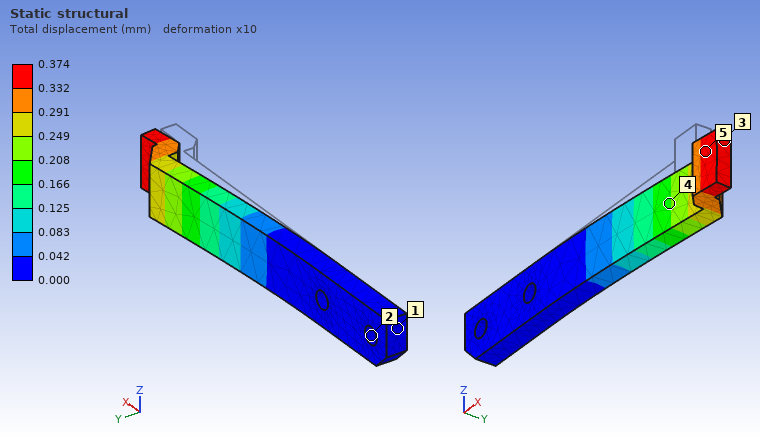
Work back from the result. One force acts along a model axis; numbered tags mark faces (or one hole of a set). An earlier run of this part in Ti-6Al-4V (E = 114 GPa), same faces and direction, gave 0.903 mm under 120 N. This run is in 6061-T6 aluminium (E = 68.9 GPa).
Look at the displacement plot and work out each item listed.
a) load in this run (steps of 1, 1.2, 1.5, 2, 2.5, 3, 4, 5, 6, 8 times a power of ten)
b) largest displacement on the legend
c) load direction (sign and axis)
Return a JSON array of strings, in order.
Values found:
["30 N", "0.374 mm", "+Y"]
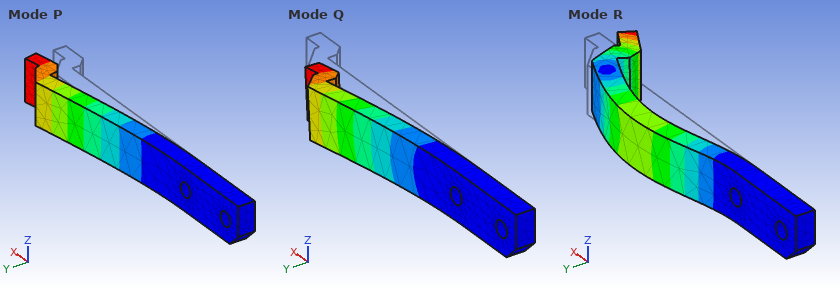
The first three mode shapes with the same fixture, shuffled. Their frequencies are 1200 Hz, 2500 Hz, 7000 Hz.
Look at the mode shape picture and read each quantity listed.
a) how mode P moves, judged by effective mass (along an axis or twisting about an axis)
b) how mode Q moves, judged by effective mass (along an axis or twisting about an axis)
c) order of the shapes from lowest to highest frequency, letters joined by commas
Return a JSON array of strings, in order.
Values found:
["along Y", "along Z", "P, Q, R"]
